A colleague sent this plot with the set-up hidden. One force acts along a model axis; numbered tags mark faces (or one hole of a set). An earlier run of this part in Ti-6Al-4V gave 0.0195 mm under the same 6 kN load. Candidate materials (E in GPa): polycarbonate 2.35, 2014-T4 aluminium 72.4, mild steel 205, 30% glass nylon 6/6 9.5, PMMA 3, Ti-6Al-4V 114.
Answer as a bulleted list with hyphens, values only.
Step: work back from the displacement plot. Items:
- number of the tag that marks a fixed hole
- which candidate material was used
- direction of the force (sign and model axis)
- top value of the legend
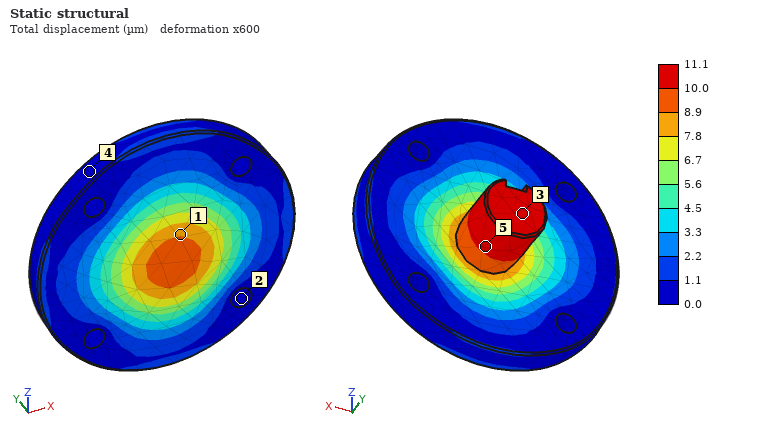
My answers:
- 2
- mild steel
- -Y
- 11.1 µm
